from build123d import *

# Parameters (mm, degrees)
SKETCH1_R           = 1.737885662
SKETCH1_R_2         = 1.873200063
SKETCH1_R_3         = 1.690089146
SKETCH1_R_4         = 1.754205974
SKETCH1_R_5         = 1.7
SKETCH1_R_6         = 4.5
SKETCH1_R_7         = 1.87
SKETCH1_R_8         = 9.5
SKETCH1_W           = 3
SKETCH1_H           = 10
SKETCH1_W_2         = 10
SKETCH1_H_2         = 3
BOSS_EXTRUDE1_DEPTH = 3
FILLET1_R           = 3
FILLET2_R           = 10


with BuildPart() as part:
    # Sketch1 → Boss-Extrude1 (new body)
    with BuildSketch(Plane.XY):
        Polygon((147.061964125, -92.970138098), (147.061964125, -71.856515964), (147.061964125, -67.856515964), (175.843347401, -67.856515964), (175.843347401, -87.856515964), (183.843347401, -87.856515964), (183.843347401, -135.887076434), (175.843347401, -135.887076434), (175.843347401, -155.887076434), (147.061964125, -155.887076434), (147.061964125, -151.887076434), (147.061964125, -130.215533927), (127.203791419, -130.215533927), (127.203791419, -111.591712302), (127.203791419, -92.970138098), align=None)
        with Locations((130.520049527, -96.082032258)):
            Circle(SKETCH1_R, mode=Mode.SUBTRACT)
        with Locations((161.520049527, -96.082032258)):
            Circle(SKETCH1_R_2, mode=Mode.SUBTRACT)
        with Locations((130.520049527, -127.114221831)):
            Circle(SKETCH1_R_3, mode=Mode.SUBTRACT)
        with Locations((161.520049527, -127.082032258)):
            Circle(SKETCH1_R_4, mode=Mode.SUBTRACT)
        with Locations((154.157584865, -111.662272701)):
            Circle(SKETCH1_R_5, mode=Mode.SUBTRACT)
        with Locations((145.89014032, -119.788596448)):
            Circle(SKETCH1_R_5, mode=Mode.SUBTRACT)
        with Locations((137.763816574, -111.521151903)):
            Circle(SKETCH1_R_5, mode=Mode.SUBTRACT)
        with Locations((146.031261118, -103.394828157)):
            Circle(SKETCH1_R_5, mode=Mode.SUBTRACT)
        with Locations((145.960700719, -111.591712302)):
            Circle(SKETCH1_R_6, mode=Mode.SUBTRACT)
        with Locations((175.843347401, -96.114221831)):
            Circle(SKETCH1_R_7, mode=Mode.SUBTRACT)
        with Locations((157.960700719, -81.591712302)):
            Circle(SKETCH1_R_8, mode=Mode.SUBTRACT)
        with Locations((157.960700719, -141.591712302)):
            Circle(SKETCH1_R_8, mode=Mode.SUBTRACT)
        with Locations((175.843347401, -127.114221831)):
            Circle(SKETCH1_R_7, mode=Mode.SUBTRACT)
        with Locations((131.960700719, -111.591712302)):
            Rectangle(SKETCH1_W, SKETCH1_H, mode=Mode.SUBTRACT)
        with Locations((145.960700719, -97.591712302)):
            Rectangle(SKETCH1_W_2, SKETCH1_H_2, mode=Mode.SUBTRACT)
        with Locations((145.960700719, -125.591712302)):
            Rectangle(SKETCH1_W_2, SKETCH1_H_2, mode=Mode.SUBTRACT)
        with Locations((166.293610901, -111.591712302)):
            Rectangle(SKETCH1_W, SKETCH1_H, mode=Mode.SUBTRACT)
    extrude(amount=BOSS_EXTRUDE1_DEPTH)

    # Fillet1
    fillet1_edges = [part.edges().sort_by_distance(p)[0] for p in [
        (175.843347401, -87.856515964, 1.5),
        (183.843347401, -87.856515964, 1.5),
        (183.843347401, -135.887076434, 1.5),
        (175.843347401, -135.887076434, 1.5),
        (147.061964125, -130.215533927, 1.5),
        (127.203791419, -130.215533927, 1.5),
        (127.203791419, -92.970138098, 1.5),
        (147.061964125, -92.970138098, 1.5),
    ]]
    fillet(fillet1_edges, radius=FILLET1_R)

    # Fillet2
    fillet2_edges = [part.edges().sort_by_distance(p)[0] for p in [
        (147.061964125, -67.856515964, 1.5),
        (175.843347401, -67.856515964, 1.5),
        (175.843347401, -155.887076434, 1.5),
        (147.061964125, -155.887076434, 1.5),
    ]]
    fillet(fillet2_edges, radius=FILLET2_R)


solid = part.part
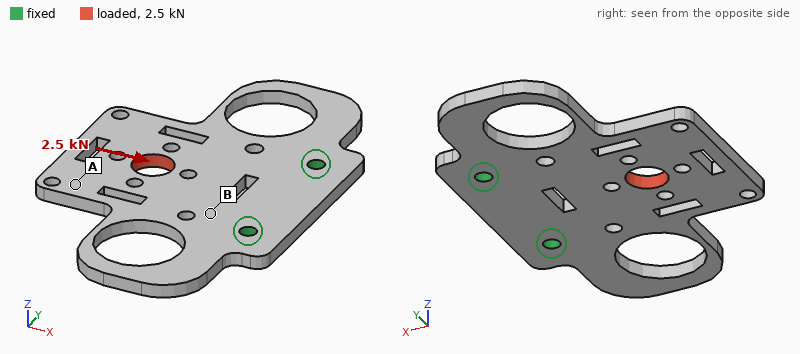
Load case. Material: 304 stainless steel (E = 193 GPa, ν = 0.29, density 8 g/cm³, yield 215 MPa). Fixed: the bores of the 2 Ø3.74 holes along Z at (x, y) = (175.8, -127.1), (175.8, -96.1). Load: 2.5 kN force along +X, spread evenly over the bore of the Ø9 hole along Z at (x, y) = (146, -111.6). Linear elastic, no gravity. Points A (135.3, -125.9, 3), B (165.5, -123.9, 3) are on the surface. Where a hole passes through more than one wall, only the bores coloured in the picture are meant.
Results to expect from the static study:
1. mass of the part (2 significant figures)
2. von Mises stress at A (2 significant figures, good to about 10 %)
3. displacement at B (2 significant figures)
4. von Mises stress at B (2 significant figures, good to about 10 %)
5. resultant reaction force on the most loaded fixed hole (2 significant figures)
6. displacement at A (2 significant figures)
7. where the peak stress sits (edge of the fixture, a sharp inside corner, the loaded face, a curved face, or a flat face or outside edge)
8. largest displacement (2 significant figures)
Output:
65 g
12 MPa
1.8 µm
32 MPa
1.3 kN
4.3 µm
a curved face
7.7 µm
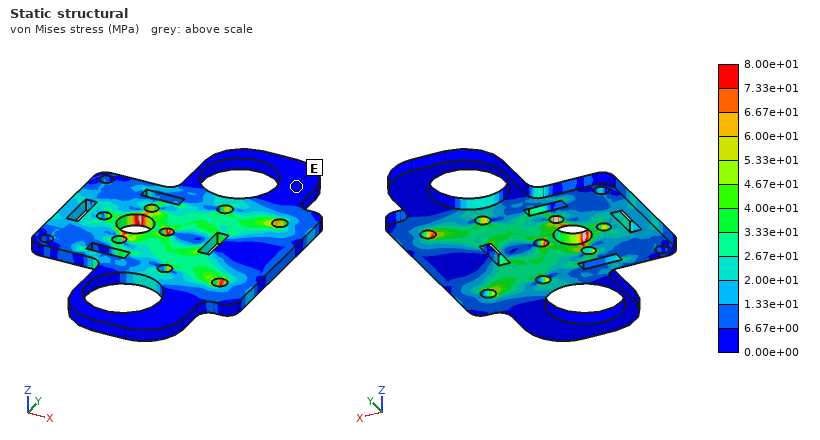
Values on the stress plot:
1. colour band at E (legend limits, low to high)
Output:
0.00e+00 to 6.67e+00 MPa
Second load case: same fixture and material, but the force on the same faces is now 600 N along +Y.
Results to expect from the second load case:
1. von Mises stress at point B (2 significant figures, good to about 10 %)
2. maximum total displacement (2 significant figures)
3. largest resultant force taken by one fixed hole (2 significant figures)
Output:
14 MPa
7.5 µm
610 N
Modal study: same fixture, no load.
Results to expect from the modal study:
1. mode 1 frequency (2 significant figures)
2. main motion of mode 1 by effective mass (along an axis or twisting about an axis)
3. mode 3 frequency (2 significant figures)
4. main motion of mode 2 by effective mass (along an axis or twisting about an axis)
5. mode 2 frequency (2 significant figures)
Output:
1100 Hz
along Z
2600 Hz
twisting about X
2300 Hz
